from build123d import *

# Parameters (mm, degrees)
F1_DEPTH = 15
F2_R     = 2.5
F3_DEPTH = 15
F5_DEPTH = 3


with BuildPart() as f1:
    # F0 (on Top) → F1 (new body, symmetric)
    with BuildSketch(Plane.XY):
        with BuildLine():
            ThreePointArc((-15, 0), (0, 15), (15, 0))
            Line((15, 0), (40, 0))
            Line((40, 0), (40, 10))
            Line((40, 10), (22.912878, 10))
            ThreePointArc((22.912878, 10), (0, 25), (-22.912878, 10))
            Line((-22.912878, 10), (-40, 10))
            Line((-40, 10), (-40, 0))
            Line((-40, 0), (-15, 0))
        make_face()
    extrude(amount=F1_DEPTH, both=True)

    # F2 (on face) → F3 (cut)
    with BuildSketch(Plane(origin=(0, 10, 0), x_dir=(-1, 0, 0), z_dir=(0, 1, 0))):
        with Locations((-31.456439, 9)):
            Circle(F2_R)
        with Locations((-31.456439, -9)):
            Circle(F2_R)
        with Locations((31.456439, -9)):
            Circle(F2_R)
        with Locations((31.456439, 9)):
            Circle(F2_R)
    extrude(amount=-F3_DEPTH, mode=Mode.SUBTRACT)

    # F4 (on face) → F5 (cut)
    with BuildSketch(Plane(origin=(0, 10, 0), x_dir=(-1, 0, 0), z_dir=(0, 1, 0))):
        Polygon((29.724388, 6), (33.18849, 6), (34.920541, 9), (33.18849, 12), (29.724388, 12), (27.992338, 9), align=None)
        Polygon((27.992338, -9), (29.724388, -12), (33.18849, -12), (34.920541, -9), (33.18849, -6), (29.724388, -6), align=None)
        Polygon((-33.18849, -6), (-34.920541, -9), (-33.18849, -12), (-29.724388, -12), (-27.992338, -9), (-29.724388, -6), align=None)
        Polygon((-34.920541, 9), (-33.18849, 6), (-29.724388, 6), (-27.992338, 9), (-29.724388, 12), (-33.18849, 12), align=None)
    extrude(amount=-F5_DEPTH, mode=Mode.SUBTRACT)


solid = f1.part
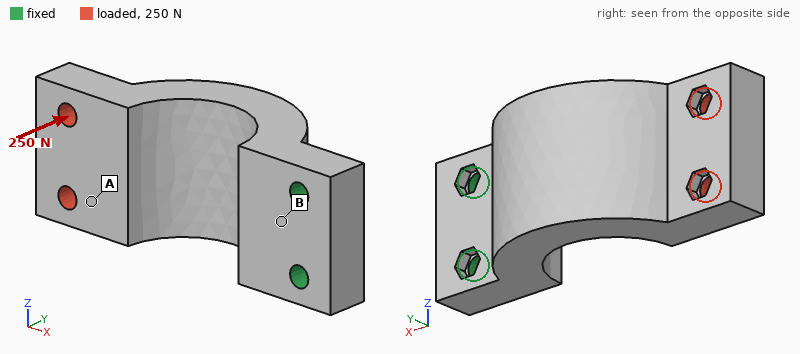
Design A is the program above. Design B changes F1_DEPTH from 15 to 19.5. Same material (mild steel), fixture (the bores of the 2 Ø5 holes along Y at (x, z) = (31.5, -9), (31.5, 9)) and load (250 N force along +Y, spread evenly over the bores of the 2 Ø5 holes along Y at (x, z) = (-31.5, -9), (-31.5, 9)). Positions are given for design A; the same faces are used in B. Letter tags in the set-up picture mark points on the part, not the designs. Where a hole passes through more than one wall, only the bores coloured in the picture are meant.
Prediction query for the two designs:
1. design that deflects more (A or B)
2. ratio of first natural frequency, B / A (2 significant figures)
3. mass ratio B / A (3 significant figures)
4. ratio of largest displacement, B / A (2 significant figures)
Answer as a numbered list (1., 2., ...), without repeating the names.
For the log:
1. A
2. 0.97
3. 1.31
4. 0.80
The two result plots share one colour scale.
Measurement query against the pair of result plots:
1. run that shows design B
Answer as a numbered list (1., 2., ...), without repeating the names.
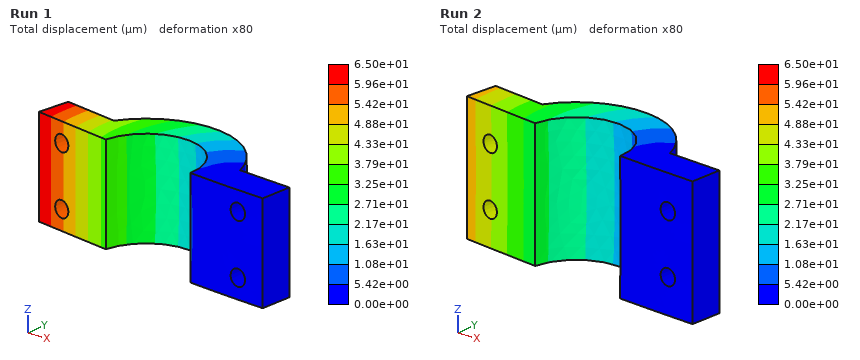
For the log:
1. Run 2
